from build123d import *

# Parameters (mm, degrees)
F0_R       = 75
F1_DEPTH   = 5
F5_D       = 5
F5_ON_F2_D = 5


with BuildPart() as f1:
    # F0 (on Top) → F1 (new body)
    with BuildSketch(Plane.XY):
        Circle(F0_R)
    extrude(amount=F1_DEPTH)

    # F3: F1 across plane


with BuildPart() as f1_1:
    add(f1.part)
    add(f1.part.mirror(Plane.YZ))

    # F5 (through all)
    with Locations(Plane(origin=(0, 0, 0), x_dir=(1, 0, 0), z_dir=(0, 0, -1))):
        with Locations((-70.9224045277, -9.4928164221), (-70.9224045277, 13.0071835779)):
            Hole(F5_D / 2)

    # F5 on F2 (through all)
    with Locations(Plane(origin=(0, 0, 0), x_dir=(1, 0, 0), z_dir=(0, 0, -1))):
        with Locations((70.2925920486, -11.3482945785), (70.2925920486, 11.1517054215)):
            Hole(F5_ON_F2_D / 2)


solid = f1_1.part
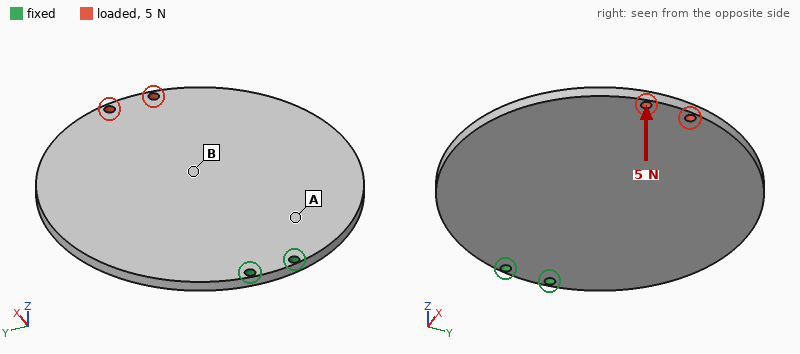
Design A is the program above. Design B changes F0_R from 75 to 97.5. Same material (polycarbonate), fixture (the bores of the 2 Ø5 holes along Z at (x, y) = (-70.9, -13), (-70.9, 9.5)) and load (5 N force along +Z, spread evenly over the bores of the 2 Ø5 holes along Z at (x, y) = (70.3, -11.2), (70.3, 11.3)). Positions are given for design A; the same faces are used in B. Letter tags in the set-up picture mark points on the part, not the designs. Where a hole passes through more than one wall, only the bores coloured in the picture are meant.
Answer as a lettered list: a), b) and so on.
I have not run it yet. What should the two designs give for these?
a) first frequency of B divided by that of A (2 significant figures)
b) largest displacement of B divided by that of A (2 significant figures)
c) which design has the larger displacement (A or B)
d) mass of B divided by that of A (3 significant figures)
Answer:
a) 0.82
b) 0.84
c) A
d) 1.69
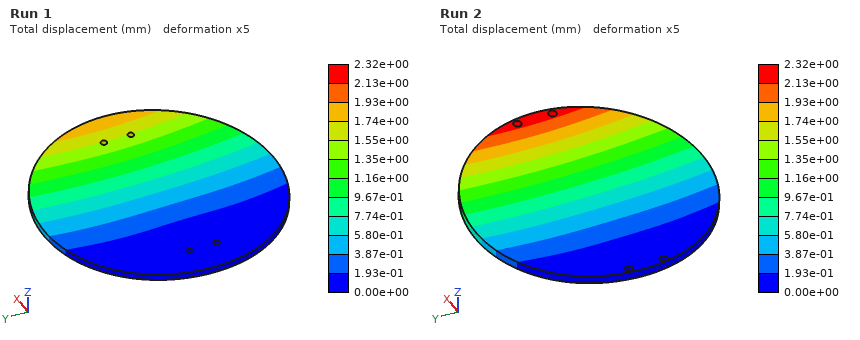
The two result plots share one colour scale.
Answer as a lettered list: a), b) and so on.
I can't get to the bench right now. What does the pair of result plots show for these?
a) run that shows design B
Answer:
a) Run 1
